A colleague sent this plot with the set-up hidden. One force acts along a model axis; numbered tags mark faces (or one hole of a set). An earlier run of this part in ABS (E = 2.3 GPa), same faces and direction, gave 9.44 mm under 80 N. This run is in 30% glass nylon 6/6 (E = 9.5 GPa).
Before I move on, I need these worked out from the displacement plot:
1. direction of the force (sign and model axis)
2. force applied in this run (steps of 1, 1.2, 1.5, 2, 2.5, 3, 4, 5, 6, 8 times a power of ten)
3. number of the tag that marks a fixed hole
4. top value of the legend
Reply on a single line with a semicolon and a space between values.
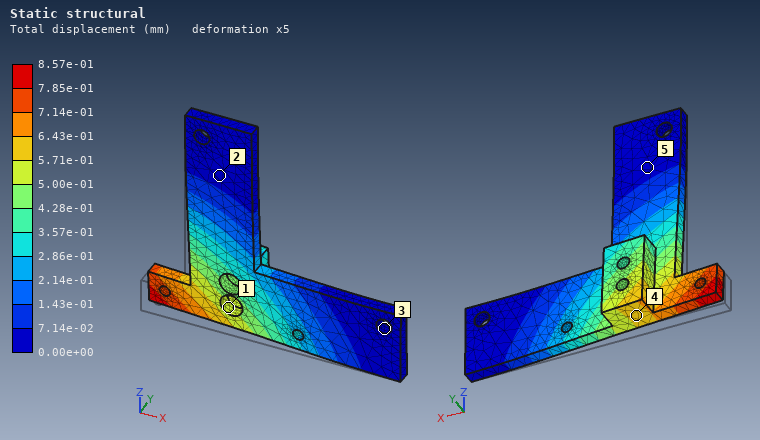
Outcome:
+Y; 30 N; 3; 8.57e-01 mm
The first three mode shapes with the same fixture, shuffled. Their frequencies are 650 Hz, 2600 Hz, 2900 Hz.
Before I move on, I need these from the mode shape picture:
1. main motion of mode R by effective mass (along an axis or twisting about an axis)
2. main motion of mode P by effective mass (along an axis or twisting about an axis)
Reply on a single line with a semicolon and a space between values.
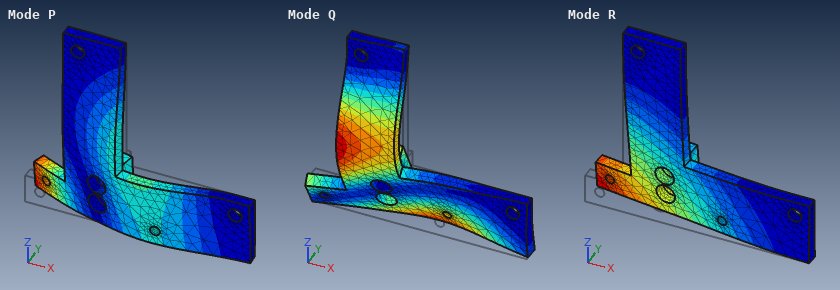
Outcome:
along Y; along Y
